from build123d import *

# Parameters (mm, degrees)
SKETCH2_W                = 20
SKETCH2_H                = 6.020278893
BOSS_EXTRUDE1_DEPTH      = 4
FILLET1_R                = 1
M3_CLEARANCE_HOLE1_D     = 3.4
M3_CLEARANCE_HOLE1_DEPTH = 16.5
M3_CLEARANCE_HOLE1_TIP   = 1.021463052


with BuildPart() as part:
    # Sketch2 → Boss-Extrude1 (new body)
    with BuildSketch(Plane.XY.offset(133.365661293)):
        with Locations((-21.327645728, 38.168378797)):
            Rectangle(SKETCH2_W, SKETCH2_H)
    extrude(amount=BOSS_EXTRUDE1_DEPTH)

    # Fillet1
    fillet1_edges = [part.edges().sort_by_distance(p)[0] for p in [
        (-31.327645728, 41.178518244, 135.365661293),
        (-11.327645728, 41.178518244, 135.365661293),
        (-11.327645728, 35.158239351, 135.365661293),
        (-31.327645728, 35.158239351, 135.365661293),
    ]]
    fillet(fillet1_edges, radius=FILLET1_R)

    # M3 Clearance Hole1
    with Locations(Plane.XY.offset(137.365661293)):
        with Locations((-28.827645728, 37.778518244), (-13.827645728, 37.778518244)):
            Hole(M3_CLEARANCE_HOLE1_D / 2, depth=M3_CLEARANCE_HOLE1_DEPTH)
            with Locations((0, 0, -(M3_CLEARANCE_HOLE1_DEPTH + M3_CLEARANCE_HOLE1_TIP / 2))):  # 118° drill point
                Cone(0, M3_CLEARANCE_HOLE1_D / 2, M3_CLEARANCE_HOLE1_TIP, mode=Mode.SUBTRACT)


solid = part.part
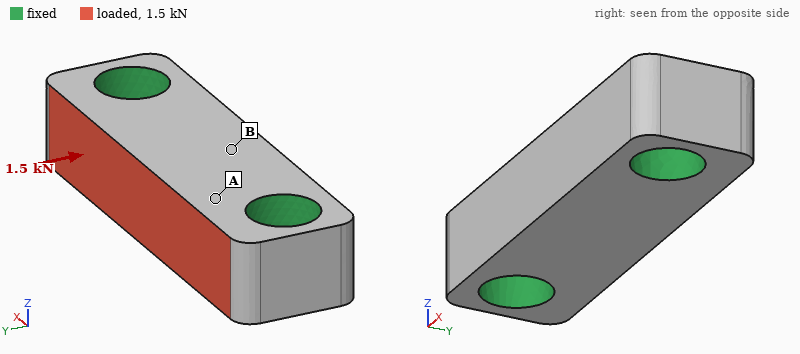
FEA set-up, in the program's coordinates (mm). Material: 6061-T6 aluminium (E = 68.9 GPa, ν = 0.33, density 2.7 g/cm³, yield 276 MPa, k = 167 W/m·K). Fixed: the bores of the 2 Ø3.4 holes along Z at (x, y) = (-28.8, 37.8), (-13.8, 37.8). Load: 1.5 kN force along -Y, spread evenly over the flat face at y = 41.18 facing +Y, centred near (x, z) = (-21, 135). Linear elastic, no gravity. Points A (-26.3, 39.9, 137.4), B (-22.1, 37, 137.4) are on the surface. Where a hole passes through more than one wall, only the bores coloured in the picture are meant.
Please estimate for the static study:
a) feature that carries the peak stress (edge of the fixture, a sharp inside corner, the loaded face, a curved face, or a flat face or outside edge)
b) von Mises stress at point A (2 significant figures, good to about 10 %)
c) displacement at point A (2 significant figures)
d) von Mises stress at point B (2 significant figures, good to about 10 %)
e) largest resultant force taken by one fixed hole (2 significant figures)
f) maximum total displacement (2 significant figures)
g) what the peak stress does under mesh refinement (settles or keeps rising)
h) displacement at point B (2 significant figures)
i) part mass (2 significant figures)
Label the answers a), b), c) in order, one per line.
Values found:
a) edge of the fixture
b) 34 MPa
c) 2.0 µm
d) 11 MPa
e) 760 N
f) 5.4 µm
g) keeps rising
h) 4.7 µm
i) 1.1 g
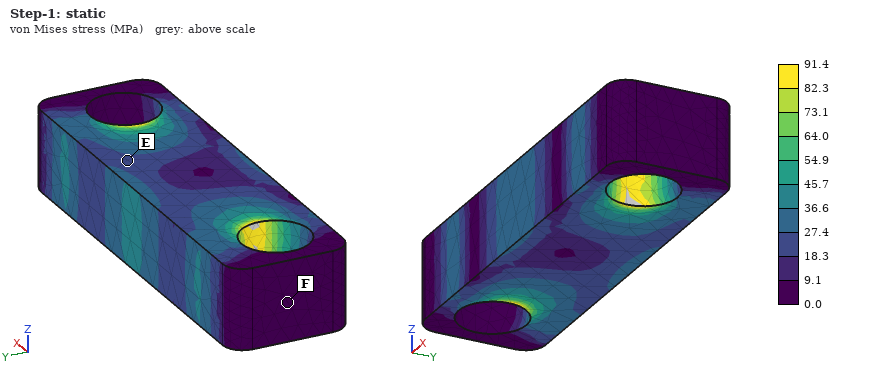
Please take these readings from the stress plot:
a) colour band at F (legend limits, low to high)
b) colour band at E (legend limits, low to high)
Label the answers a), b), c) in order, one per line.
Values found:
a) 0.0 to 9.1 MPa
b) 18.3 to 27.4 MPa
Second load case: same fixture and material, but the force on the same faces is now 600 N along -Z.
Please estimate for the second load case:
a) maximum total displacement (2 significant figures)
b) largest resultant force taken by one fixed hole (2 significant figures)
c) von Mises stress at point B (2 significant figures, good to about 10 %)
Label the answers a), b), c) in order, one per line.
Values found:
a) 7.0 µm
b) 300 N
c) 12 MPa
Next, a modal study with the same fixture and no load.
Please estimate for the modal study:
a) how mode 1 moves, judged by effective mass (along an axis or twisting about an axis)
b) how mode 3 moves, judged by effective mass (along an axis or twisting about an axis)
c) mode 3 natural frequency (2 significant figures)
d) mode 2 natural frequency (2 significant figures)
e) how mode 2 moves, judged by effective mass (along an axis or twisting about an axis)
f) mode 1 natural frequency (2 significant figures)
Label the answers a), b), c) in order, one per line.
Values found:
a) along Z
b) twisting about X
c) 110 kHz
d) 91 kHz
e) along Y
f) 85 kHz
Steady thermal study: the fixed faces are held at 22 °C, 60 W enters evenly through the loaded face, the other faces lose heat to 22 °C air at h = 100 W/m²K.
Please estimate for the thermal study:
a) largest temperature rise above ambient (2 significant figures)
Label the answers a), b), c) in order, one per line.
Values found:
a) 28 K
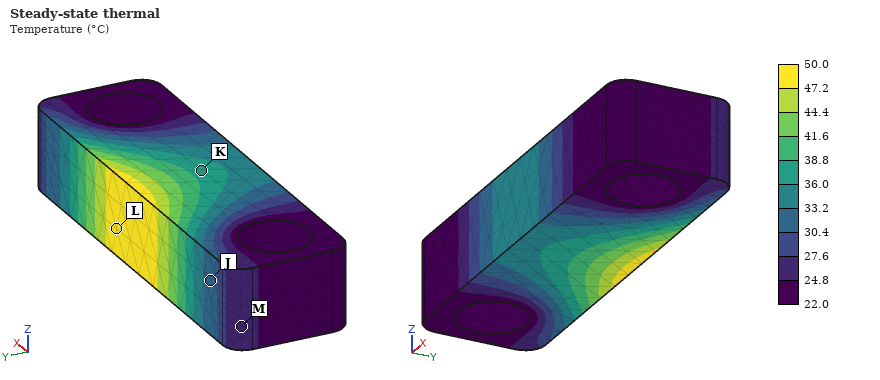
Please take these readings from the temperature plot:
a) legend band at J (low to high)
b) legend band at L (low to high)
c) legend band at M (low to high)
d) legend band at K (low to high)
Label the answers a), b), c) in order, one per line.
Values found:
a) 30.4 to 33.2 °C
b) 47.2 to 50.0 °C
c) 24.8 to 27.6 °C
d) 36.0 to 38.8 °C
